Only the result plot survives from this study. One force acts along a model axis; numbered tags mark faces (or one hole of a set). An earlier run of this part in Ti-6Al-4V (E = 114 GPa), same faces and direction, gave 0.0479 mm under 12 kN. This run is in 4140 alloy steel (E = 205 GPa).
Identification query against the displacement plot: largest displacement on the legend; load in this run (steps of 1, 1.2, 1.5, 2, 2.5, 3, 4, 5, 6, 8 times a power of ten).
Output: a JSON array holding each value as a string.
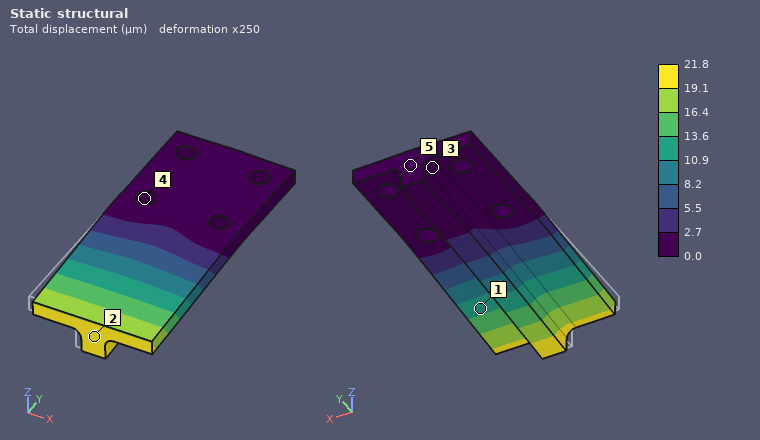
["21.8 µm", "10 kN"]
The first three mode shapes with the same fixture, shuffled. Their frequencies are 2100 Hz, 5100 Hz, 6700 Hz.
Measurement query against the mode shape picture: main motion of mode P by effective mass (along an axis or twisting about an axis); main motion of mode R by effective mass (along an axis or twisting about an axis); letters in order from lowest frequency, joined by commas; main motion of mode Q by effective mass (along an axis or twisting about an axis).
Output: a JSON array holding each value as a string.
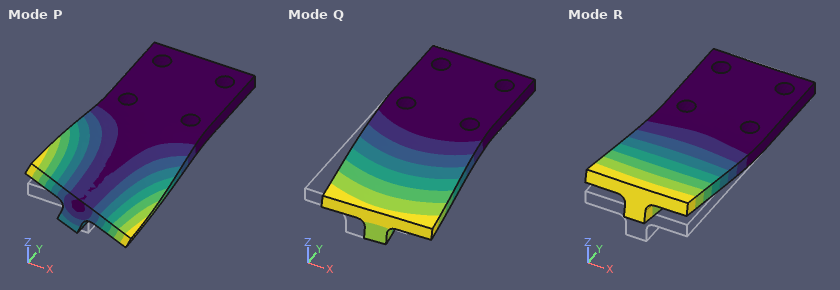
["twisting about Y", "along Z", "R, P, Q", "along X"]
